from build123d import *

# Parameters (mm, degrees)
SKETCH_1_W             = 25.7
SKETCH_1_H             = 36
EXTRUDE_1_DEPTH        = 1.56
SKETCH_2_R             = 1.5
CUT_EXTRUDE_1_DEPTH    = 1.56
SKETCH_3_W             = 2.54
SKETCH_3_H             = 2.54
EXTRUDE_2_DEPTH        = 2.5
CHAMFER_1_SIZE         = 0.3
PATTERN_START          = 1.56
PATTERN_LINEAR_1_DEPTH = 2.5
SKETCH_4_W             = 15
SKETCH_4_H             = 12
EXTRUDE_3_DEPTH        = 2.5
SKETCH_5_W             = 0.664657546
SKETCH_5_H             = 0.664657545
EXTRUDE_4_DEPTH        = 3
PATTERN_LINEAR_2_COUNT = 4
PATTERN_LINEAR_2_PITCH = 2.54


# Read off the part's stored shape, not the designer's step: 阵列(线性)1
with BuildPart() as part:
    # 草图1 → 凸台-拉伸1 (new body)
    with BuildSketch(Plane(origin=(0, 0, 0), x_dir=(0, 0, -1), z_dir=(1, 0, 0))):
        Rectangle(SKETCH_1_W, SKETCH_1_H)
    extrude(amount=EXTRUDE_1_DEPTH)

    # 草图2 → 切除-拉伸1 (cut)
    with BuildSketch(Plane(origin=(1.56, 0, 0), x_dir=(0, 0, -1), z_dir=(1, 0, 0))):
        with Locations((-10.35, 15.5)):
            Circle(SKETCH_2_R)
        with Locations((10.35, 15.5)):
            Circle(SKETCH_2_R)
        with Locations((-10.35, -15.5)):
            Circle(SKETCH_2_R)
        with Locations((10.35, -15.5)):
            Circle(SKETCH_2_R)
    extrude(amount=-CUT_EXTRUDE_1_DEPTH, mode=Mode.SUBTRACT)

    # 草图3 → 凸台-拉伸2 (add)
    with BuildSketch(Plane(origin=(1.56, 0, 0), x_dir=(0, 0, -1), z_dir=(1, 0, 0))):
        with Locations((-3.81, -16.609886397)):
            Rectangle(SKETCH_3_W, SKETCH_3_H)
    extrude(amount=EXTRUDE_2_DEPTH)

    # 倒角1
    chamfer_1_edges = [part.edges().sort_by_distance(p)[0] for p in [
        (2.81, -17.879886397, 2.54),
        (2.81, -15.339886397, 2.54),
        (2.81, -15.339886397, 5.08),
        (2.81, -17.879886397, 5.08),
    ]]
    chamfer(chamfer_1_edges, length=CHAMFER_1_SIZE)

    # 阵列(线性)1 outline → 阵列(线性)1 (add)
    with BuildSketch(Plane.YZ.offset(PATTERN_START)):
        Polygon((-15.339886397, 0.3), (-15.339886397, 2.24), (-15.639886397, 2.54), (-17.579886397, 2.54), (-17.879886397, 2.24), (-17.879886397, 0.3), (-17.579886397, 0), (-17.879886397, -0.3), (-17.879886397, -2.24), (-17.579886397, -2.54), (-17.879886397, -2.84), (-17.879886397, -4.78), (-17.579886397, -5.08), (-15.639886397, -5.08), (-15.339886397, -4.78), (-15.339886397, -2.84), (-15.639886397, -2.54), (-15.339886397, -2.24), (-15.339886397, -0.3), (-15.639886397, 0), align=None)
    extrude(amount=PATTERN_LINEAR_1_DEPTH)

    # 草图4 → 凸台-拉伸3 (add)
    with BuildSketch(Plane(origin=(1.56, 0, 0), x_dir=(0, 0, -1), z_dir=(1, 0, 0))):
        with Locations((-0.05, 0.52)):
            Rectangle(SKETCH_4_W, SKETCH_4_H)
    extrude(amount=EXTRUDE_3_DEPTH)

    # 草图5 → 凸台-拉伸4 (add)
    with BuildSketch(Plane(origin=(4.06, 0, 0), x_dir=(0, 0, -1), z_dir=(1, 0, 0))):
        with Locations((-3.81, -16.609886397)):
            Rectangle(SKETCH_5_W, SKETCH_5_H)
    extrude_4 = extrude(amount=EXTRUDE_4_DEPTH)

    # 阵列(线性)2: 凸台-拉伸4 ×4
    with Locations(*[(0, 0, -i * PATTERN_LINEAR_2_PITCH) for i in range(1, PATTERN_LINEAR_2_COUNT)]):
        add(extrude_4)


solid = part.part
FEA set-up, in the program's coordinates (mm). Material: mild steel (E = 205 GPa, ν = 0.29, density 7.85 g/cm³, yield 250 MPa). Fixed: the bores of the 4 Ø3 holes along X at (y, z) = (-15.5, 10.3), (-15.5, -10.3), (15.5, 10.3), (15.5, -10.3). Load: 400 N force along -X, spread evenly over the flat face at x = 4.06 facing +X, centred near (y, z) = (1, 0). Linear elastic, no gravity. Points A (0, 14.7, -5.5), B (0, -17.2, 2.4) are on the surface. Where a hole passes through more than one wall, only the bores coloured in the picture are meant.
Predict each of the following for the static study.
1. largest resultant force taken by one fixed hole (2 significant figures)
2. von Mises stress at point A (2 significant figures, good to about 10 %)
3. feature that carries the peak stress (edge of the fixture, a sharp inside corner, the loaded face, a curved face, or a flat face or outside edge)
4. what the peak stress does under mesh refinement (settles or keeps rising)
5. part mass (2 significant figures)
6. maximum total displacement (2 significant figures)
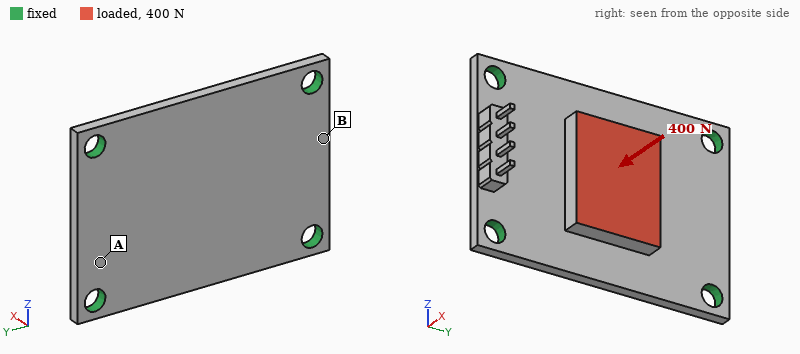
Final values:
120 N
44 MPa
edge of the fixture
keeps rising
15 g
18 µm
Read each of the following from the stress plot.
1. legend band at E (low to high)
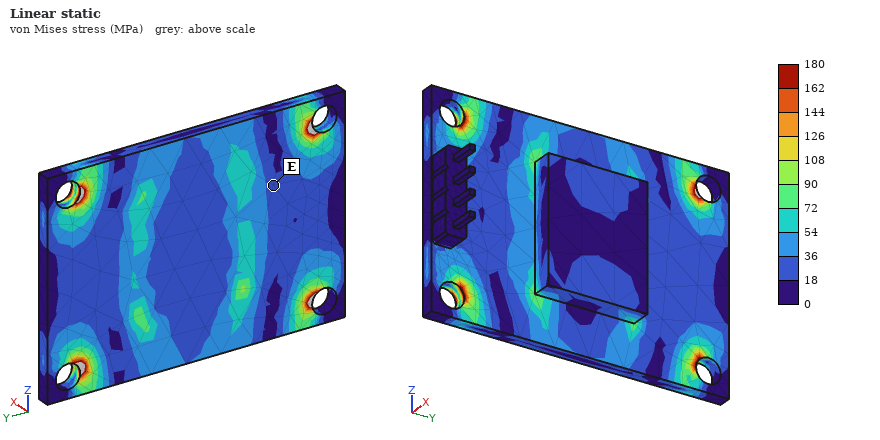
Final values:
18 to 36 MPa
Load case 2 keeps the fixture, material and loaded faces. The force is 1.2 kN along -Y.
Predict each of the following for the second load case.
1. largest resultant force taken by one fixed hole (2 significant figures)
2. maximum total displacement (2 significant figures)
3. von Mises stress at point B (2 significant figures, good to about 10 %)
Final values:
330 N
11 µm
15 MPa
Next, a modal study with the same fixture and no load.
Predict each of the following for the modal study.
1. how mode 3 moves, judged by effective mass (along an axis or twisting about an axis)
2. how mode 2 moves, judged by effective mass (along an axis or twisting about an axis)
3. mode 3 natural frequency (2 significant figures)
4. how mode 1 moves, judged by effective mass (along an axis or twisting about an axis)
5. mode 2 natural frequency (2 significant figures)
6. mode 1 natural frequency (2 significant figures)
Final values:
twisting about Z
twisting about Y
19 kHz
along X
12 kHz
8100 Hz
